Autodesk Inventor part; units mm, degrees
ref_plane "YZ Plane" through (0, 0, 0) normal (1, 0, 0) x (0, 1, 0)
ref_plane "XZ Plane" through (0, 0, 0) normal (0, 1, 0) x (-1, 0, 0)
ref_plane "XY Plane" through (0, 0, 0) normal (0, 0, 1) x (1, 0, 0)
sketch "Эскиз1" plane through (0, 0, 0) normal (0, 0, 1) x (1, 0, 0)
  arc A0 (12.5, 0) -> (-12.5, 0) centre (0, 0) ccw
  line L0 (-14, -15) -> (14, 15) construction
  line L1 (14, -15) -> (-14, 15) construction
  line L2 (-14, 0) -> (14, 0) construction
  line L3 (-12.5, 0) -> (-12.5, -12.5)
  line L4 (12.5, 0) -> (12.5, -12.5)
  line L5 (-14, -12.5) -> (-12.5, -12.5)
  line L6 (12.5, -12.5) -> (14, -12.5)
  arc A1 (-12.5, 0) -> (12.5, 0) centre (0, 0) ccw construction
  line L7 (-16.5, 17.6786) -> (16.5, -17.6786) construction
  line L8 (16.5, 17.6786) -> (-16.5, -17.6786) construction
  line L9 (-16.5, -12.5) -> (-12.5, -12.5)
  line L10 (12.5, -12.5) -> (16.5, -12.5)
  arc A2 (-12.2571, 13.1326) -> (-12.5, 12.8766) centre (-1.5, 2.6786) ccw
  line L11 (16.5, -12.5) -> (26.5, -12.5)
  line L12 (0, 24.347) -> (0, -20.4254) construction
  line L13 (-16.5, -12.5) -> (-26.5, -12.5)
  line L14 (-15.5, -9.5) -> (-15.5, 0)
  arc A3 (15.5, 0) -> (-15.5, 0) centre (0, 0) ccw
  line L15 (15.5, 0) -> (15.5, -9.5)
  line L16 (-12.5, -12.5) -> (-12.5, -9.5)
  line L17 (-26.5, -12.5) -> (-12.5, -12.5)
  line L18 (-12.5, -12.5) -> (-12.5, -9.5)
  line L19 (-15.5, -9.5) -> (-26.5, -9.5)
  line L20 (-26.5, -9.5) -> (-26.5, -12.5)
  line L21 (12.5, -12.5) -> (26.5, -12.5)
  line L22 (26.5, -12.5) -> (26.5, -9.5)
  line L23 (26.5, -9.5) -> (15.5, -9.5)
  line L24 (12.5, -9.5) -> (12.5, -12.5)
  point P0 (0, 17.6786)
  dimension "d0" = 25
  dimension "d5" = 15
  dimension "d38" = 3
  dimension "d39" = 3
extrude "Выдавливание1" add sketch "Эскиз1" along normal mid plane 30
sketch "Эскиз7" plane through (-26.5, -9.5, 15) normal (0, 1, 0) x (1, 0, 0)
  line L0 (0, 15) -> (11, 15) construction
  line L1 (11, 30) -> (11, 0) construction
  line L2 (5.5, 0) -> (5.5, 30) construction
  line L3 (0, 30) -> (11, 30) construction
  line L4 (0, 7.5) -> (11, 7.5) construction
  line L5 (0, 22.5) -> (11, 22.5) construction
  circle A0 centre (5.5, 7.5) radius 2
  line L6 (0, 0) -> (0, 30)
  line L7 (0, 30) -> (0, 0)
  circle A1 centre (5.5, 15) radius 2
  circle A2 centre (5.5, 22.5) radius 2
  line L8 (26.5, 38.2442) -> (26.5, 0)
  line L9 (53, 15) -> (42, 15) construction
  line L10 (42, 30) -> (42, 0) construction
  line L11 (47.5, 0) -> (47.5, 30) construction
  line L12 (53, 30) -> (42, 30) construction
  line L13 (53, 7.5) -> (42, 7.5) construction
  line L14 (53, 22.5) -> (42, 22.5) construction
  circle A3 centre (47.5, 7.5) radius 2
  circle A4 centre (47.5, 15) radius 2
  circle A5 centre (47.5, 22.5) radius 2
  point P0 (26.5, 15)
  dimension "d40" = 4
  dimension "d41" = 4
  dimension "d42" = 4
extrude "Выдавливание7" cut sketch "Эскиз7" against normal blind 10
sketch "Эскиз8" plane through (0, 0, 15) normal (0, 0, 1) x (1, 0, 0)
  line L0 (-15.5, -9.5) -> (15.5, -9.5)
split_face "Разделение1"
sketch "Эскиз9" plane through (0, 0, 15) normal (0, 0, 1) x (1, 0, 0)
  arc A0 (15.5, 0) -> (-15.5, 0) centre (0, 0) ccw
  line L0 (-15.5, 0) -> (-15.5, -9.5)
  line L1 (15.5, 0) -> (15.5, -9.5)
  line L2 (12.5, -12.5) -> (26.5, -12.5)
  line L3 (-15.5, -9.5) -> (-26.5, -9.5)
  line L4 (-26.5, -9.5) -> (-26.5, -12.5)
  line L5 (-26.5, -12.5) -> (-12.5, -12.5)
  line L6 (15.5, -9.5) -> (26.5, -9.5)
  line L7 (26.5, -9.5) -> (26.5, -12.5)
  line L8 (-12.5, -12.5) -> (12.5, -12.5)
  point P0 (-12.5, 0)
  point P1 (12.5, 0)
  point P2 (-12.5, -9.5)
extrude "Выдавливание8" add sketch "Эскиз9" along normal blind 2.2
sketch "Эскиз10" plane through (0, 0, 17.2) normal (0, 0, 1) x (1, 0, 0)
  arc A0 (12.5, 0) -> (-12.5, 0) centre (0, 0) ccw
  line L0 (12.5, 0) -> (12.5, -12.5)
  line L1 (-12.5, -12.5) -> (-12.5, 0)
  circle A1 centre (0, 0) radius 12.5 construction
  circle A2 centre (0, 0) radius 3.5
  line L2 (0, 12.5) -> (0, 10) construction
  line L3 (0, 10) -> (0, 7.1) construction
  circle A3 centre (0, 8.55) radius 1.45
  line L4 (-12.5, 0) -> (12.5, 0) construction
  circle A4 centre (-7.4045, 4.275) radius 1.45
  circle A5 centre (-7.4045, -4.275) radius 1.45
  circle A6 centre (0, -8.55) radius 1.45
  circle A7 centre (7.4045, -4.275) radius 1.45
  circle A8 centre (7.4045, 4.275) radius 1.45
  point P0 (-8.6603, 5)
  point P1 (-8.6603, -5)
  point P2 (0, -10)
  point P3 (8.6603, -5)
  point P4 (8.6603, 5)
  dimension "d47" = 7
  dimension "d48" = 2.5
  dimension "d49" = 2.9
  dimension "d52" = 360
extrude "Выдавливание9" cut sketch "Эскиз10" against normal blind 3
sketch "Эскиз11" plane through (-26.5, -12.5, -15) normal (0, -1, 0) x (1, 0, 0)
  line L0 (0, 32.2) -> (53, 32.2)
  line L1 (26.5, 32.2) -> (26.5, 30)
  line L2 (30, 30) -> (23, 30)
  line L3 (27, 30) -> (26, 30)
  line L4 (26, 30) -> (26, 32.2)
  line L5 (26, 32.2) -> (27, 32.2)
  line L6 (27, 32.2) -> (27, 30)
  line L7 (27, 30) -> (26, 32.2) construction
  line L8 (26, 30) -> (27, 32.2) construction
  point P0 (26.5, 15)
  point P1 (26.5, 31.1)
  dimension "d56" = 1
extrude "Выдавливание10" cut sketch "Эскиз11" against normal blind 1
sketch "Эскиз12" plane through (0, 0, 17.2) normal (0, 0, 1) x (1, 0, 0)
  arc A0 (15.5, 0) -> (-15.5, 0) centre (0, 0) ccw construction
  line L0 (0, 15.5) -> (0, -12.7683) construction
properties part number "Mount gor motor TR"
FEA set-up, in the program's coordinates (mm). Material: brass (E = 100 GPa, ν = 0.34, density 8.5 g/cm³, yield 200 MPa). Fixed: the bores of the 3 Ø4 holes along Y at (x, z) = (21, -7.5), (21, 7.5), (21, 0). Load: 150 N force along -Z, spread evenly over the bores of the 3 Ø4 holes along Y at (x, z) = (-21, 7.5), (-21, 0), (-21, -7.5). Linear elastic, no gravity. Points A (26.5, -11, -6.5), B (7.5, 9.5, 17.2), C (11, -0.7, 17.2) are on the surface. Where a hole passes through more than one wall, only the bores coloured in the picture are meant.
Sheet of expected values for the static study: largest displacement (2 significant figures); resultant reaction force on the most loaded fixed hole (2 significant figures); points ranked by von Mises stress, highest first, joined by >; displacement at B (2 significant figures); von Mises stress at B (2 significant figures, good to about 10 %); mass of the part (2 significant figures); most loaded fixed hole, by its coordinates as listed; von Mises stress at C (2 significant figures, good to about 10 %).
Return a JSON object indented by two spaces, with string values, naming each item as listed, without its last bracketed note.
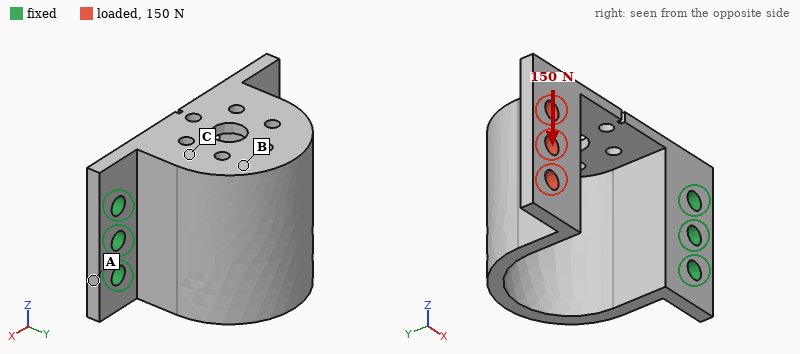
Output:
{
  "largest displacement": "0.39 mm",
  "resultant reaction force on the most loaded fixed hole": "350 N",
  "points ranked by von Mises stress, highest first, joined by >": "C > B > A",
  "displacement at B": "0.091 mm",
  "von Mises stress at B": "33 MPa",
  "mass of the part": "82 g",
  "most loaded fixed hole, by its coordinates as listed": "(21, 7.5)",
  "von Mises stress at C": "52 MPa"
}
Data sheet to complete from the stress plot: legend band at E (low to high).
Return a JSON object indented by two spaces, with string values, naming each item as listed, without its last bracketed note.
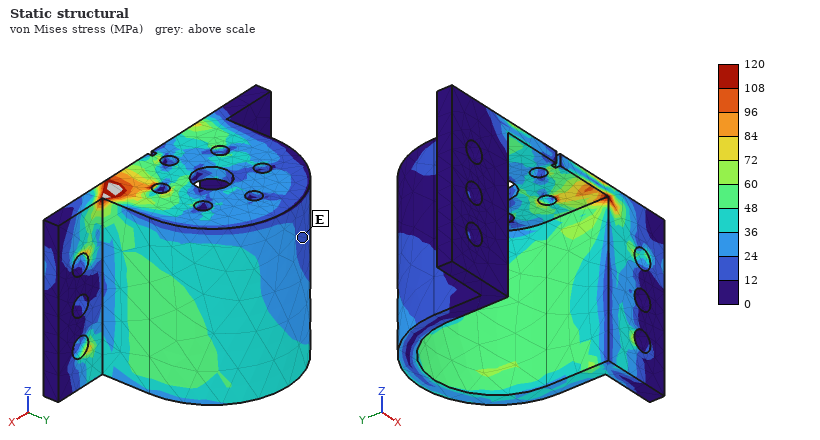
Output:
{
  "legend band at E": "12 to 24 MPa"
}
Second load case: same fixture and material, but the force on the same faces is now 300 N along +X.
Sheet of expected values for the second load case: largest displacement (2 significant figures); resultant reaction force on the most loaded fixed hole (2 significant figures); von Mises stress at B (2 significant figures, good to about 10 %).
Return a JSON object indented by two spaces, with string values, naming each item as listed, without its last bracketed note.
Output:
{
  "largest displacement": "0.46 mm",
  "resultant reaction force on the most loaded fixed hole": "160 N",
  "von Mises stress at B": "28 MPa"
}
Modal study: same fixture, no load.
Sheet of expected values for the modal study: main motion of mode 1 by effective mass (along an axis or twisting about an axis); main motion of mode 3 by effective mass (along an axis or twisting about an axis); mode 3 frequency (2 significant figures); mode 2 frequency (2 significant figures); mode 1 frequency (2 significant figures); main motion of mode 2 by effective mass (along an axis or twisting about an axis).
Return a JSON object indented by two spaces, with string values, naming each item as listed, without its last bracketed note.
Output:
{
  "main motion of mode 1 by effective mass": "along Y",
  "main motion of mode 3 by effective mass": "along X",
  "mode 3 frequency": "1700 Hz",
  "mode 2 frequency": "750 Hz",
  "mode 1 frequency": "540 Hz",
  "main motion of mode 2 by effective mass": "along Z"
}
